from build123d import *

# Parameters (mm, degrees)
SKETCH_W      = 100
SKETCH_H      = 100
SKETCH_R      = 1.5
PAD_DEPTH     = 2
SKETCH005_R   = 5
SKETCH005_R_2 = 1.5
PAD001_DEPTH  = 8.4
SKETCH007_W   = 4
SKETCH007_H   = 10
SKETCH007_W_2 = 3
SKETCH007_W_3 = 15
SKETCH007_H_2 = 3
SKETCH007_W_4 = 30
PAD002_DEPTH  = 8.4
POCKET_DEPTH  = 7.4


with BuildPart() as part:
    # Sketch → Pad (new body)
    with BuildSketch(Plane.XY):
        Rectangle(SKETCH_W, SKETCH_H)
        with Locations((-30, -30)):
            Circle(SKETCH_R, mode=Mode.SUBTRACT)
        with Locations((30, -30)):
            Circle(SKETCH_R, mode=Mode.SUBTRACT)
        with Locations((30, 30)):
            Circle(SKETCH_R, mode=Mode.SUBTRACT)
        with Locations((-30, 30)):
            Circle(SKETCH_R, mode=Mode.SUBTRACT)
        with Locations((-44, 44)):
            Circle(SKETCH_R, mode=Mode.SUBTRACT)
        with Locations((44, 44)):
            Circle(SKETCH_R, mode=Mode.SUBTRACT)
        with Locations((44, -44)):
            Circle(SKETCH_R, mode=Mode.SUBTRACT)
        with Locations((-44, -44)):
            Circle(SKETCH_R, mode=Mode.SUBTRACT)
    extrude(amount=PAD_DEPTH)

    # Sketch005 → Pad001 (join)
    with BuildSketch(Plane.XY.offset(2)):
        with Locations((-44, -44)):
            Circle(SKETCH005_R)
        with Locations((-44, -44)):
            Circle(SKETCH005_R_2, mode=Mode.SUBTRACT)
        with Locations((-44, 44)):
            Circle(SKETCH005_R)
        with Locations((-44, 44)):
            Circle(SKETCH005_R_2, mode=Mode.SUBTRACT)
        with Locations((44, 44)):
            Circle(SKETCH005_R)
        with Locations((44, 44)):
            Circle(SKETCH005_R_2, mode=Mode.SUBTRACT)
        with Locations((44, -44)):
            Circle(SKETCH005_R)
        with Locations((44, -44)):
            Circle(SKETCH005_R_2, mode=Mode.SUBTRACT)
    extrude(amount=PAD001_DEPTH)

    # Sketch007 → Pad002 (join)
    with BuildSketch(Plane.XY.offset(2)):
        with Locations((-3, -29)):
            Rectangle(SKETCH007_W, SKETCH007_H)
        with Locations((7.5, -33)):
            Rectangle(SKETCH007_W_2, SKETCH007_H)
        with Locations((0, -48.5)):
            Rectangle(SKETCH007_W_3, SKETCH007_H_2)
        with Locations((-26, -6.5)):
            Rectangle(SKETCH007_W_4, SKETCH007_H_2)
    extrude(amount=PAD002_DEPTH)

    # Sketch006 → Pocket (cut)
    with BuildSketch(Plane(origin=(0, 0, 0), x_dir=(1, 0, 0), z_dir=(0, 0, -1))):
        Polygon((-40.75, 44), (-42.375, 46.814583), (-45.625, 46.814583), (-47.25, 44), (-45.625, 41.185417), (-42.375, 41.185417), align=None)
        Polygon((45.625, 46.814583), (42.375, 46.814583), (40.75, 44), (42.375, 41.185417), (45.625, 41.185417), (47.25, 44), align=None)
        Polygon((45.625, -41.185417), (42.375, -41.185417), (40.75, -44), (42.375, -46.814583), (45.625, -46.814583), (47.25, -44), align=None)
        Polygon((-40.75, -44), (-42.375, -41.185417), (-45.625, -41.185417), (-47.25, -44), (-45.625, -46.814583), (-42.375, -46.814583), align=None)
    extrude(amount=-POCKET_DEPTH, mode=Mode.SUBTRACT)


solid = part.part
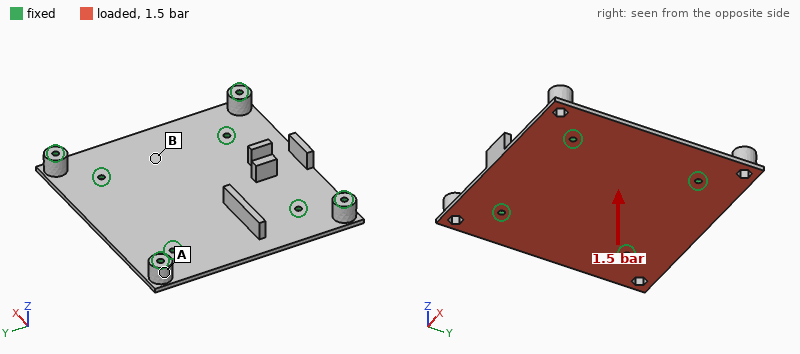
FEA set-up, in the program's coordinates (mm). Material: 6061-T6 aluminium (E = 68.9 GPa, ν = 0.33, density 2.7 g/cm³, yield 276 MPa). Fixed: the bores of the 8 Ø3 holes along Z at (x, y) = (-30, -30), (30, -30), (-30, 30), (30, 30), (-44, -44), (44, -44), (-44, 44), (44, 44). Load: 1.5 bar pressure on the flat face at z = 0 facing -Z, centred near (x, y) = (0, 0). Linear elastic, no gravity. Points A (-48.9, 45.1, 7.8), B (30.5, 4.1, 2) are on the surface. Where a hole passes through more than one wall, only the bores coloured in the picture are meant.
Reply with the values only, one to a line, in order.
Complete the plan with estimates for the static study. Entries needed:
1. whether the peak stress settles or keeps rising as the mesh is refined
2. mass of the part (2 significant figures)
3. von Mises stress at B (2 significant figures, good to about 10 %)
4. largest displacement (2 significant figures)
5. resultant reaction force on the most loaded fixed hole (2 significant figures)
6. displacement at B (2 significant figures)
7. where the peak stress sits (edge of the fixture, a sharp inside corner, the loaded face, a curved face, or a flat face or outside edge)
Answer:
keeps rising
63 g
40 MPa
0.23 mm
360 N
0.15 mm
edge of the fixture
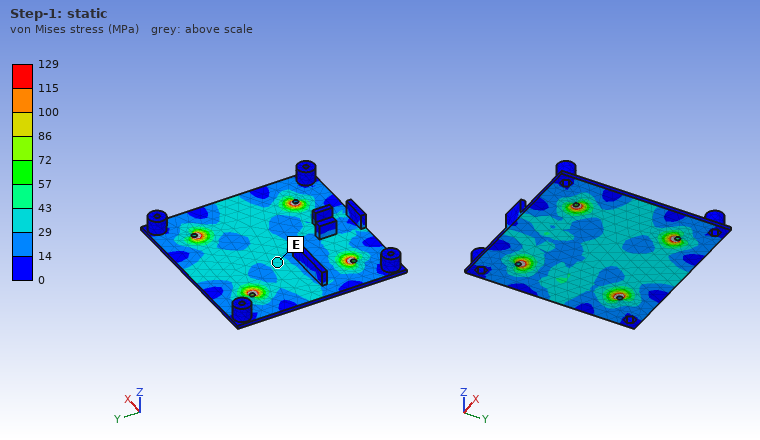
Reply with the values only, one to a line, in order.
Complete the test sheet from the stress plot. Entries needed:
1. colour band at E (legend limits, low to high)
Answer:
29 to 43 MPa
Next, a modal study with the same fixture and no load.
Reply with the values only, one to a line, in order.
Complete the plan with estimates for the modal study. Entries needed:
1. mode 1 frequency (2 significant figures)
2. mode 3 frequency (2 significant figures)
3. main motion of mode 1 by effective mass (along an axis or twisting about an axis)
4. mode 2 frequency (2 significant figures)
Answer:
2000 Hz
2400 Hz
along Z
2100 Hz
